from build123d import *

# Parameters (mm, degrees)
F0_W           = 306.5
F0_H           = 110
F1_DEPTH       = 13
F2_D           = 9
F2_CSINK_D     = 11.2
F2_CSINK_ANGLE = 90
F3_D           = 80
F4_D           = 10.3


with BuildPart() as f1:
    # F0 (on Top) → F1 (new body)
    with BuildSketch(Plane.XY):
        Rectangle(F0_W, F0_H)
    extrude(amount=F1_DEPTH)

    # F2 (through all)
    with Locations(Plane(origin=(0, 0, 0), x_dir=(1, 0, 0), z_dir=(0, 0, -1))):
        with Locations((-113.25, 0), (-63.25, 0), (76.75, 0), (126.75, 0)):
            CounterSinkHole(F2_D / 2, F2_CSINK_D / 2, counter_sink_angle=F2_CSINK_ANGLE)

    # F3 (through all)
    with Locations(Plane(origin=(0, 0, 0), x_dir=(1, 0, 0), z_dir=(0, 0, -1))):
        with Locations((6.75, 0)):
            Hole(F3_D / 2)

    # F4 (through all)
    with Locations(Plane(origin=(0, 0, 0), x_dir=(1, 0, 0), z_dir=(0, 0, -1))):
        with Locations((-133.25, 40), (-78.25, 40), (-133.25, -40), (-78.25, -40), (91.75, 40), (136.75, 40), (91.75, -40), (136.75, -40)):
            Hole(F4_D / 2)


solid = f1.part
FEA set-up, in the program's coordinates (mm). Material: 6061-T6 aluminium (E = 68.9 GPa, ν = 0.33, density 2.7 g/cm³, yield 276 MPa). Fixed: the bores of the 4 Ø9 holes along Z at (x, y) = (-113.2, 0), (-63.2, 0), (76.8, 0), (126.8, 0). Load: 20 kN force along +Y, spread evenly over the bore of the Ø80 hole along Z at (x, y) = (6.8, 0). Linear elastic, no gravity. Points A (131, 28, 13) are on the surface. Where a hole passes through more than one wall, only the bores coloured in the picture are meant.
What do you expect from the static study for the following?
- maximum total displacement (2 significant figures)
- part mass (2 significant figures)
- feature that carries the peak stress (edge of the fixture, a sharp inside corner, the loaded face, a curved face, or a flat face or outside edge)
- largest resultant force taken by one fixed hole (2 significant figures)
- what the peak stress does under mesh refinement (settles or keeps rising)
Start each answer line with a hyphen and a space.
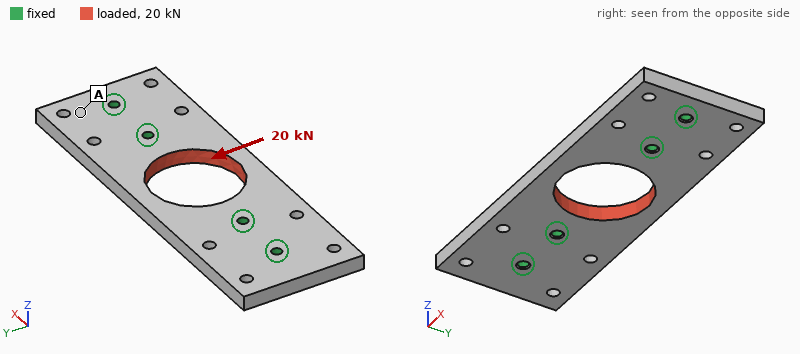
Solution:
- 38 µm
- 970 g
- edge of the fixture
- 11 kN
- keeps rising
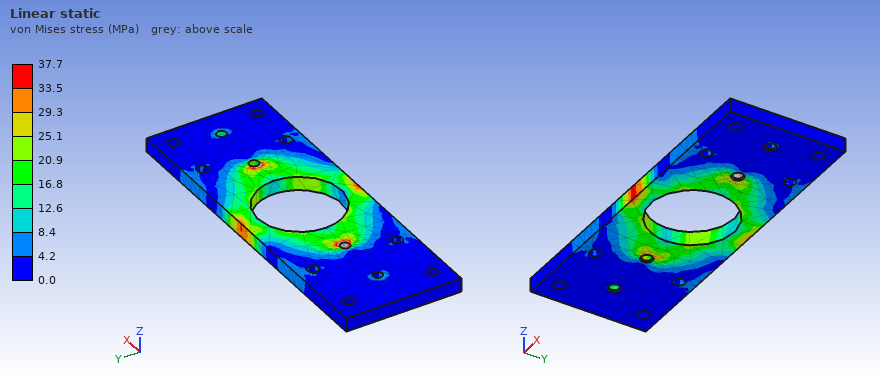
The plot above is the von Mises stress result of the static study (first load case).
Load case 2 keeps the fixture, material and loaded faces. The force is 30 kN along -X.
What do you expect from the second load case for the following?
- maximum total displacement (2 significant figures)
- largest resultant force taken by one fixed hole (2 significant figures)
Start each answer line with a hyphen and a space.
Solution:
- 22 µm
- 10.0 kN
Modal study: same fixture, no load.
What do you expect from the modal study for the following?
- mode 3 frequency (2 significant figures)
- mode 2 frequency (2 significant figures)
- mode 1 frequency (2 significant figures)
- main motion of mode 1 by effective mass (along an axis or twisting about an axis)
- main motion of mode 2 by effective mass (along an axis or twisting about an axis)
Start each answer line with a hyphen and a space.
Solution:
- 2700 Hz
- 2600 Hz
- 2100 Hz
- twisting about X
- along Z
